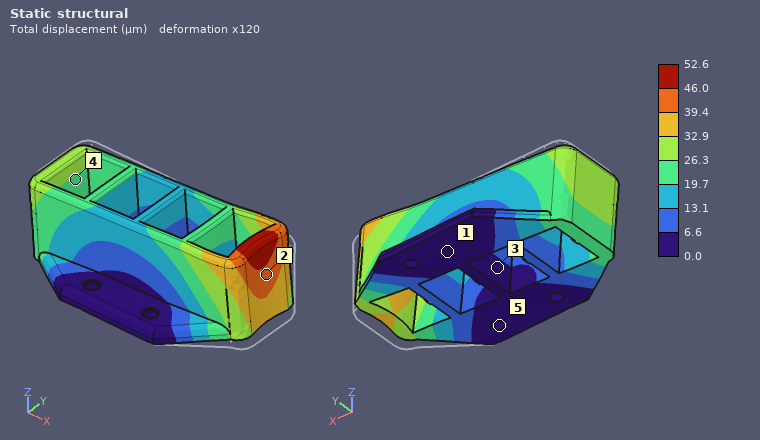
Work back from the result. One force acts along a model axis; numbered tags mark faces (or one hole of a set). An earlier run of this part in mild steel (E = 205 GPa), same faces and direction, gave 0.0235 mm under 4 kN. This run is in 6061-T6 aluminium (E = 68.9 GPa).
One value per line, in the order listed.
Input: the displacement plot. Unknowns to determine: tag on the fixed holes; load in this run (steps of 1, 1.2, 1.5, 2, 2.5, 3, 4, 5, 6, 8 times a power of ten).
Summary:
5
3 kN
